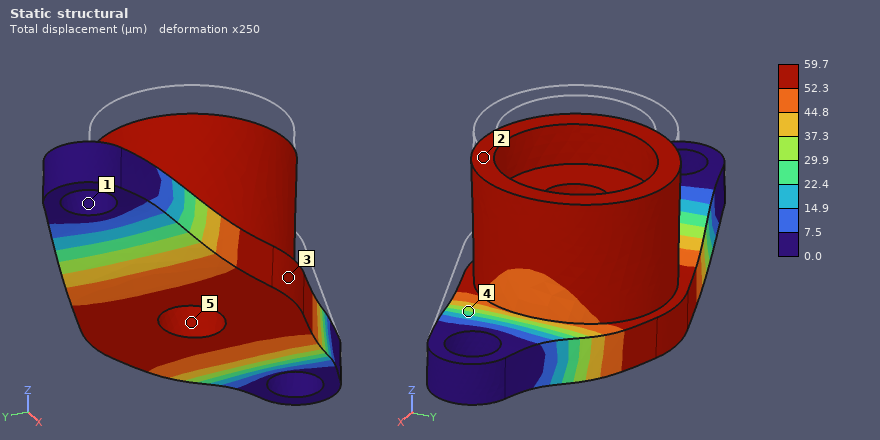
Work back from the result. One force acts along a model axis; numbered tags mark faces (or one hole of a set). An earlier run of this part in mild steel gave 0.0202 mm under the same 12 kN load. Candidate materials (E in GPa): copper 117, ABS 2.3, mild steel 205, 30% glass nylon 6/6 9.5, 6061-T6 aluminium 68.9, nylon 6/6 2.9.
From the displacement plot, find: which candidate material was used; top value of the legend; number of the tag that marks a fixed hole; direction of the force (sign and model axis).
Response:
6061-T6 aluminium
59.7 µm
1
-Z
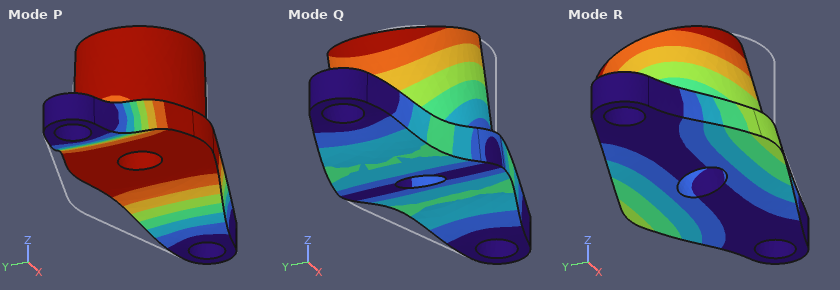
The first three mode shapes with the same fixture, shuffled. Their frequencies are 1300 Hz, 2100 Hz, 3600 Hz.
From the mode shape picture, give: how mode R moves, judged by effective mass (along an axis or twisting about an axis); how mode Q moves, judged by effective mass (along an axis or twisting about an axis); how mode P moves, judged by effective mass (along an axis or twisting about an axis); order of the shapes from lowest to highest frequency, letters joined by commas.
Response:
along Y
along X
along Z
R, P, Q
